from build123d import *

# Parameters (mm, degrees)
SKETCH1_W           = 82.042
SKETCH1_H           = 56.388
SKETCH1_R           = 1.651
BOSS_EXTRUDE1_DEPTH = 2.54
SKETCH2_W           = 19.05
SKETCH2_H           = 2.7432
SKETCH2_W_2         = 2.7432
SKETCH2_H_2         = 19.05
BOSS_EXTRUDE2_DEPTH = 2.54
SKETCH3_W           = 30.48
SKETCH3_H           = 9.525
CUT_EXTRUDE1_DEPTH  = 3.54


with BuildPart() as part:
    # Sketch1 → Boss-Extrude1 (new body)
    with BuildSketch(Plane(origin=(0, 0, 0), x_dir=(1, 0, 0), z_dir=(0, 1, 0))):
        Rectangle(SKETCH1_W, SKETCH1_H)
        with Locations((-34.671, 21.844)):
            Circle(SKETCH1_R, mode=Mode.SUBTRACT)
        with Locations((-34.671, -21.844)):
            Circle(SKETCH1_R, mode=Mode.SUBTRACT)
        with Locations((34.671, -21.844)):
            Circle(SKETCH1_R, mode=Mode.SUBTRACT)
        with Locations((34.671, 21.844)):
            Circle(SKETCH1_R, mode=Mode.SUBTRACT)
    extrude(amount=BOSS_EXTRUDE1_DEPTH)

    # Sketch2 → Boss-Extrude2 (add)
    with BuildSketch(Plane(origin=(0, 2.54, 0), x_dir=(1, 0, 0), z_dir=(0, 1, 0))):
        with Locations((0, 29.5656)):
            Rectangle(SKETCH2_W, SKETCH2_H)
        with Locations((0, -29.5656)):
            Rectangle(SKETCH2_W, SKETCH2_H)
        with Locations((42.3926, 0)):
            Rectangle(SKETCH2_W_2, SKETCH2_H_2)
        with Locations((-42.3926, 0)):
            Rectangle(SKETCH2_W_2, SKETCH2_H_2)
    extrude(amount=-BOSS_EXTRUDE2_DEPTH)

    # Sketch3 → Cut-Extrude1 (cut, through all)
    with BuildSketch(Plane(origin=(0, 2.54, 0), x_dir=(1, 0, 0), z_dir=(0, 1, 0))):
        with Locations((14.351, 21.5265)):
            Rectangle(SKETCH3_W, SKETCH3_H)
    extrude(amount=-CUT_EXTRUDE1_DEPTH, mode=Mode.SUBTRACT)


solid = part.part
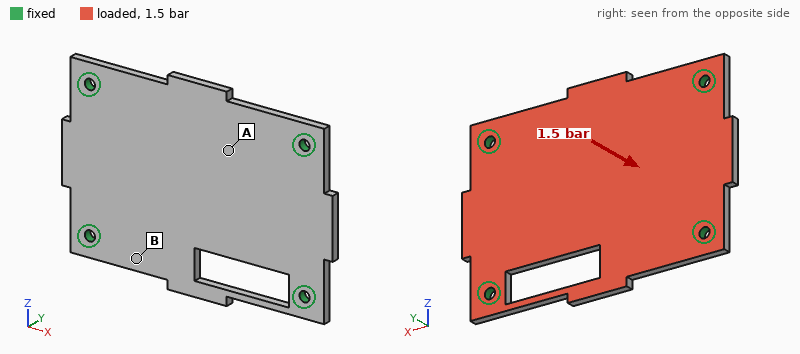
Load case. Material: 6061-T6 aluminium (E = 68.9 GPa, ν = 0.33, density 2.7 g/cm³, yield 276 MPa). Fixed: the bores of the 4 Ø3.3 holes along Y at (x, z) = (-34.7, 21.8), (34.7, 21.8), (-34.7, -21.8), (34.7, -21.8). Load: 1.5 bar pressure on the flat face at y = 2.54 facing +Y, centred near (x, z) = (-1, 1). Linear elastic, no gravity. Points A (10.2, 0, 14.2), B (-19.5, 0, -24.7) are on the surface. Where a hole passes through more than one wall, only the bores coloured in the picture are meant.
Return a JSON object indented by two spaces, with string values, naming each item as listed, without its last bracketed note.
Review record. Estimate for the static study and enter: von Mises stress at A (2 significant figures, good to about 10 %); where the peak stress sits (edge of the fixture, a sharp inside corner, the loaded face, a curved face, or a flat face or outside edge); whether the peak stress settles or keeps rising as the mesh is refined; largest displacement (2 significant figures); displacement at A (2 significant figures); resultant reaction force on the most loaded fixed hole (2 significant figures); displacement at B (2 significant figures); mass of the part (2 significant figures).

{
  "von Mises stress at A": "24 MPa",
  "where the peak stress sits": "edge of the fixture",
  "whether the peak stress settles or keeps rising as the mesh is refined": "keeps rising",
  "largest displacement": "0.14 mm",
  "displacement at A": "0.11 mm",
  "resultant reaction force on the most loaded fixed hole": "180 N",
  "displacement at B": "0.059 mm",
  "mass of the part": "31 g"
}
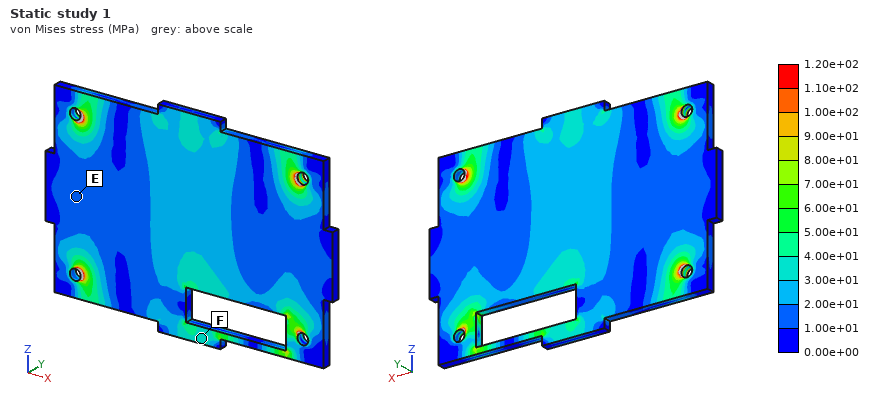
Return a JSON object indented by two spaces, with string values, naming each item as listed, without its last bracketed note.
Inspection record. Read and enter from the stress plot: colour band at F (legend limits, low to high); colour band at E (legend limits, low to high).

{
  "colour band at F": "3.00e+01 to 4.00e+01 MPa",
  "colour band at E": "1.00e+01 to 2.00e+01 MPa"
}
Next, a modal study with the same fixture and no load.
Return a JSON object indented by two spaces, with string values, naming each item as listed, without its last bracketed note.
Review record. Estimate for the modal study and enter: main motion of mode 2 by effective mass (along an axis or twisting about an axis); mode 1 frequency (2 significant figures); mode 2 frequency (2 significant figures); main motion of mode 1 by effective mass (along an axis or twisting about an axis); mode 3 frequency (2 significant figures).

{
  "main motion of mode 2 by effective mass": "twisting about X",
  "mode 1 frequency": "2300 Hz",
  "mode 2 frequency": "3300 Hz",
  "main motion of mode 1 by effective mass": "along Y",
  "mode 3 frequency": "4900 Hz"
}
